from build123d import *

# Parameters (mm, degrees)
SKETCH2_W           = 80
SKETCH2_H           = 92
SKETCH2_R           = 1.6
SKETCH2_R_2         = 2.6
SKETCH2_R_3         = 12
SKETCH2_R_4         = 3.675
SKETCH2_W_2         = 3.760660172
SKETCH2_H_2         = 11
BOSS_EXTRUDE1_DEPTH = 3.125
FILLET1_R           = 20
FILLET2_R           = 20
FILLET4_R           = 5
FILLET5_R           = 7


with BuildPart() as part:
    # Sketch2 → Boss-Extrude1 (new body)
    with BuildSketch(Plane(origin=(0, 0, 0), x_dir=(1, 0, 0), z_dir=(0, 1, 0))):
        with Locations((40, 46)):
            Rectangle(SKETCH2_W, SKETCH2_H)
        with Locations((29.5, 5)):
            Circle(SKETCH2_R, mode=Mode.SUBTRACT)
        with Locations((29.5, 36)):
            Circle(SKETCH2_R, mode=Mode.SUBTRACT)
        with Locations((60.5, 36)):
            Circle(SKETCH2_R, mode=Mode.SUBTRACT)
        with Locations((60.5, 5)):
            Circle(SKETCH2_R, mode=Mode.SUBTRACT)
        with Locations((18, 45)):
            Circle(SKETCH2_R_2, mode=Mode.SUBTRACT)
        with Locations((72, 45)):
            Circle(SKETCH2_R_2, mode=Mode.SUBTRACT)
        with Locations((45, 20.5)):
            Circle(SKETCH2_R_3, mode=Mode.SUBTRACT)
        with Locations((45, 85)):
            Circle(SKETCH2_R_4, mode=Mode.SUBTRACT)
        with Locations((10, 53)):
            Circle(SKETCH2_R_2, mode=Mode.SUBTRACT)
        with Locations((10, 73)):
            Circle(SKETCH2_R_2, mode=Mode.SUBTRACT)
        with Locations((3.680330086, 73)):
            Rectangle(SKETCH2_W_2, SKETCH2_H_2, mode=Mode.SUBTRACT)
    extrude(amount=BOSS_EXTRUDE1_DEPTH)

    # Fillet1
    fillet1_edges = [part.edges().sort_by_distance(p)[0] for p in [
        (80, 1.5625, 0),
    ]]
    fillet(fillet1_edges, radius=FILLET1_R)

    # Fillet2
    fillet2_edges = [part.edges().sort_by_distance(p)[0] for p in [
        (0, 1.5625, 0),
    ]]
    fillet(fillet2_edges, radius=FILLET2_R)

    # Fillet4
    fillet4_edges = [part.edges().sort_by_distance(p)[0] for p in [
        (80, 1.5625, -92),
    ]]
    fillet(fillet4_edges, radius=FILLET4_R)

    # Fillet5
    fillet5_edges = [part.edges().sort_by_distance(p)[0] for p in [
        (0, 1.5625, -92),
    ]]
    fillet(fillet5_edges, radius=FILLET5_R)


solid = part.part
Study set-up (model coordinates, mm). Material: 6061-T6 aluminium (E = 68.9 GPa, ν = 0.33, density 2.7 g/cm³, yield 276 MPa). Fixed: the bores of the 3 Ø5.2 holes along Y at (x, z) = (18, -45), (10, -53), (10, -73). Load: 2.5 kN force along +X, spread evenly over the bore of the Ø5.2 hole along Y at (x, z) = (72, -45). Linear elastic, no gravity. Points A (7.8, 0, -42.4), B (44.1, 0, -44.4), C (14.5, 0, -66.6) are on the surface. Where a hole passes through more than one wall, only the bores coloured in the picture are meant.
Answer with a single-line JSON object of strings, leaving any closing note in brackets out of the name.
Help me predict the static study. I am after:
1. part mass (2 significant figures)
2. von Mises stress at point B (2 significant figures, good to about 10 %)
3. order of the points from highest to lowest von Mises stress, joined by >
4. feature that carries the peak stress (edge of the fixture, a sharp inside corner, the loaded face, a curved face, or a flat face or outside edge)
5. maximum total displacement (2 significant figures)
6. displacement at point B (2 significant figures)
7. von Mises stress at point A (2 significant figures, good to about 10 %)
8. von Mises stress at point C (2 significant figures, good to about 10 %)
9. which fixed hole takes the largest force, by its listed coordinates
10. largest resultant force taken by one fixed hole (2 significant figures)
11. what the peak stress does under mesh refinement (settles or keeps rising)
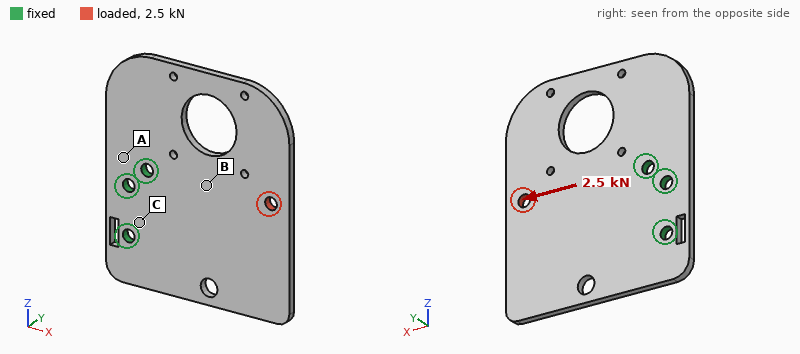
{"part mass": "55 g", "von Mises stress at point B": "26 MPa", "order of the points from highest to lowest von Mises stress, joined by >": "B > A > C", "feature that carries the peak stress": "edge of the fixture", "maximum total displacement": "36 µm", "displacement at point B": "14 µm", "von Mises stress at point A": "14 MPa", "von Mises stress at point C": "5.8 MPa", "which fixed hole takes the largest force, by its listed coordinates": "(18, -45)", "largest resultant force taken by one fixed hole": "2.0 kN", "what the peak stress does under mesh refinement": "keeps rising"}
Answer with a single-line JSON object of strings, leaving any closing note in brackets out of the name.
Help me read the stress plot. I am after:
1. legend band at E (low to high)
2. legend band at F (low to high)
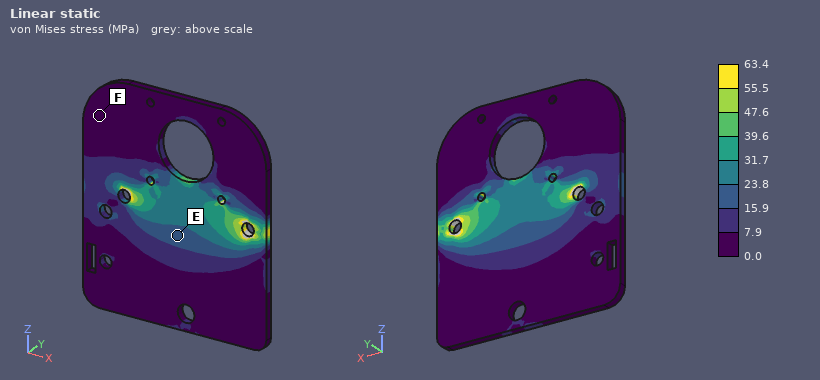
{"legend band at E": "15.9 to 23.8 MPa", "legend band at F": "0.0 to 7.9 MPa"}
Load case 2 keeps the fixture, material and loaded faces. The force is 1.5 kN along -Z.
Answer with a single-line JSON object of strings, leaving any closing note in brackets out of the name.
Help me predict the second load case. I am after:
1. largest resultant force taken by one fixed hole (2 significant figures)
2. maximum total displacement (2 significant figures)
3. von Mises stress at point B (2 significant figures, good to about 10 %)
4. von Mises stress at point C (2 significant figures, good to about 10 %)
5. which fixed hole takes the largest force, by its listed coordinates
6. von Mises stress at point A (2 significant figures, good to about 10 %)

{"largest resultant force taken by one fixed hole": "3.0 kN", "maximum total displacement": "85 µm", "von Mises stress at point B": "17 MPa", "von Mises stress at point C": "27 MPa", "which fixed hole takes the largest force, by its listed coordinates": "(18, -45)", "von Mises stress at point A": "24 MPa"}
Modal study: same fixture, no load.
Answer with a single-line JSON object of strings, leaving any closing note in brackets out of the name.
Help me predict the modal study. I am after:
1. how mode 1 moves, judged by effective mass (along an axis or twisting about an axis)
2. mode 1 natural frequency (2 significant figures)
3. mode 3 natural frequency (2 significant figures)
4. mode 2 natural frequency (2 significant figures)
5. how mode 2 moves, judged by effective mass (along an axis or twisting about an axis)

{"how mode 1 moves, judged by effective mass": "along Y", "mode 1 natural frequency": "570 Hz", "mode 3 natural frequency": "1700 Hz", "mode 2 natural frequency": "880 Hz", "how mode 2 moves, judged by effective mass": "twisting about X"}
